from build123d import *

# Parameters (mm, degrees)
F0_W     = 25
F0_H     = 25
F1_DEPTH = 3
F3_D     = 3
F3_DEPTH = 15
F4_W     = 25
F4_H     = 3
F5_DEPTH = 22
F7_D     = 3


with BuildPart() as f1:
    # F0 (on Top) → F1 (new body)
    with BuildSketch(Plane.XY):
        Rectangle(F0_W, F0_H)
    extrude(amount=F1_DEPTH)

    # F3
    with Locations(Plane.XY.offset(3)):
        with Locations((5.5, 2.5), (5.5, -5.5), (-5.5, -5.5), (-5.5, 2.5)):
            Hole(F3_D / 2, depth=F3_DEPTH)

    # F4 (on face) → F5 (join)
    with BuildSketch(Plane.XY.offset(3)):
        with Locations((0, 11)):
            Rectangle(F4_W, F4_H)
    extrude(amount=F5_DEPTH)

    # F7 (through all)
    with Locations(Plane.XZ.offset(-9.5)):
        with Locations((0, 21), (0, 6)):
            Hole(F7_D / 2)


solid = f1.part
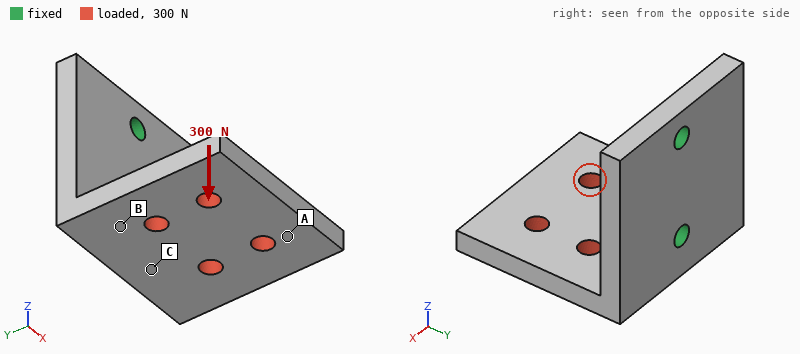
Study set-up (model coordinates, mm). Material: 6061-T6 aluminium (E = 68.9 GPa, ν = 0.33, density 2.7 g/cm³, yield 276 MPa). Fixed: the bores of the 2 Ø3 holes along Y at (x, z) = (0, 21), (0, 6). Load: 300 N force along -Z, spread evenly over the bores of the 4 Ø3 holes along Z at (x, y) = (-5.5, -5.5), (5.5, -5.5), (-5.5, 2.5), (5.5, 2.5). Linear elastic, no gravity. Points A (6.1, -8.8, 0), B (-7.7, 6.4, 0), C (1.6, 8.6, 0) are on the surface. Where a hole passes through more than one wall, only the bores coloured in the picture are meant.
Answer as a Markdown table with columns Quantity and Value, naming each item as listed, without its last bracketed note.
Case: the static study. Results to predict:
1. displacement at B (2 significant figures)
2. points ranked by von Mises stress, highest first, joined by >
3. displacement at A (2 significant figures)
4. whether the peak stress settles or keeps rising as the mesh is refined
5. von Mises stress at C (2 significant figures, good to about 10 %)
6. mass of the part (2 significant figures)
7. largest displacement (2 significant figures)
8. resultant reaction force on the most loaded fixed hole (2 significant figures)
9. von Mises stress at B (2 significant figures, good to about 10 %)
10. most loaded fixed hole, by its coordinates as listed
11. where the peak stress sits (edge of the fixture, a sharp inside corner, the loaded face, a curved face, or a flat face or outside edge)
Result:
| Quantity | Value |
|---|---|
| displacement at B | 0.038 mm |
| points ranked by von Mises stress, highest first, joined by > | C > B > A |
| displacement at A | 0.19 mm |
| whether the peak stress settles or keeps rising as the mesh is refined | keeps rising |
| von Mises stress at C | 84 MPa |
| mass of the part | 9.2 g |
| largest displacement | 0.23 mm |
| resultant reaction force on the most loaded fixed hole | 270 N |
| von Mises stress at B | 54 MPa |
| most loaded fixed hole, by its coordinates as listed | (0, 6) |
| where the peak stress sits | edge of the fixture |
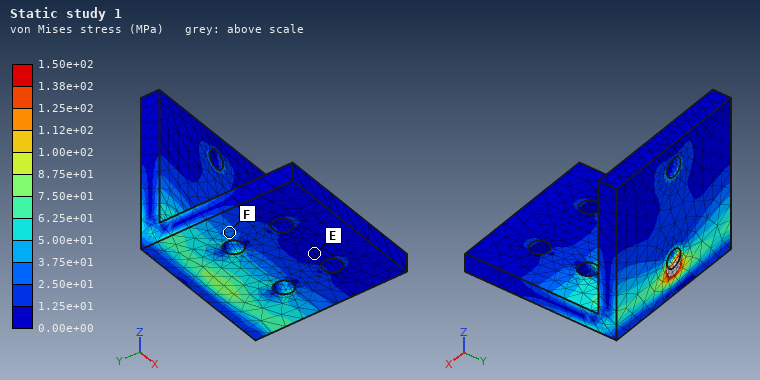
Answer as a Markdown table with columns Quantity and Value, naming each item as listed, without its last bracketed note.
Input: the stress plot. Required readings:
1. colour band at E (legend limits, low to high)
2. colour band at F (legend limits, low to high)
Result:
| Quantity | Value |
|---|---|
| colour band at E | 0.00e+00 to 1.25e+01 MPa |
| colour band at F | 2.50e+01 to 3.75e+01 MPa |
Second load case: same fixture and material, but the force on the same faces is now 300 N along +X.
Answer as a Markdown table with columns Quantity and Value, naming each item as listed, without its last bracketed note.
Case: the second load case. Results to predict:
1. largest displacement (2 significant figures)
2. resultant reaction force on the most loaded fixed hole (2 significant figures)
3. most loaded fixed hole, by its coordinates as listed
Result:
| Quantity | Value |
|---|---|
| largest displacement | 92 µm |
| resultant reaction force on the most loaded fixed hole | 360 N |
| most loaded fixed hole, by its coordinates as listed | (0, 6) |
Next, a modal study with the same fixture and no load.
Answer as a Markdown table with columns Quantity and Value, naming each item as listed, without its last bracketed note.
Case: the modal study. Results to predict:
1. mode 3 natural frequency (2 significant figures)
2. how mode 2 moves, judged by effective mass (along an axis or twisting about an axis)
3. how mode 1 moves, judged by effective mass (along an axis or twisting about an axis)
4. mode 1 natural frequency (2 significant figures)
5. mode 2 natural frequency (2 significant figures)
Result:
| Quantity | Value |
|---|---|
| mode 3 natural frequency | 8700 Hz |
| how mode 2 moves, judged by effective mass | along X |
| how mode 1 moves, judged by effective mass | along Z |
| mode 1 natural frequency | 3400 Hz |
| mode 2 natural frequency | 4900 Hz |
